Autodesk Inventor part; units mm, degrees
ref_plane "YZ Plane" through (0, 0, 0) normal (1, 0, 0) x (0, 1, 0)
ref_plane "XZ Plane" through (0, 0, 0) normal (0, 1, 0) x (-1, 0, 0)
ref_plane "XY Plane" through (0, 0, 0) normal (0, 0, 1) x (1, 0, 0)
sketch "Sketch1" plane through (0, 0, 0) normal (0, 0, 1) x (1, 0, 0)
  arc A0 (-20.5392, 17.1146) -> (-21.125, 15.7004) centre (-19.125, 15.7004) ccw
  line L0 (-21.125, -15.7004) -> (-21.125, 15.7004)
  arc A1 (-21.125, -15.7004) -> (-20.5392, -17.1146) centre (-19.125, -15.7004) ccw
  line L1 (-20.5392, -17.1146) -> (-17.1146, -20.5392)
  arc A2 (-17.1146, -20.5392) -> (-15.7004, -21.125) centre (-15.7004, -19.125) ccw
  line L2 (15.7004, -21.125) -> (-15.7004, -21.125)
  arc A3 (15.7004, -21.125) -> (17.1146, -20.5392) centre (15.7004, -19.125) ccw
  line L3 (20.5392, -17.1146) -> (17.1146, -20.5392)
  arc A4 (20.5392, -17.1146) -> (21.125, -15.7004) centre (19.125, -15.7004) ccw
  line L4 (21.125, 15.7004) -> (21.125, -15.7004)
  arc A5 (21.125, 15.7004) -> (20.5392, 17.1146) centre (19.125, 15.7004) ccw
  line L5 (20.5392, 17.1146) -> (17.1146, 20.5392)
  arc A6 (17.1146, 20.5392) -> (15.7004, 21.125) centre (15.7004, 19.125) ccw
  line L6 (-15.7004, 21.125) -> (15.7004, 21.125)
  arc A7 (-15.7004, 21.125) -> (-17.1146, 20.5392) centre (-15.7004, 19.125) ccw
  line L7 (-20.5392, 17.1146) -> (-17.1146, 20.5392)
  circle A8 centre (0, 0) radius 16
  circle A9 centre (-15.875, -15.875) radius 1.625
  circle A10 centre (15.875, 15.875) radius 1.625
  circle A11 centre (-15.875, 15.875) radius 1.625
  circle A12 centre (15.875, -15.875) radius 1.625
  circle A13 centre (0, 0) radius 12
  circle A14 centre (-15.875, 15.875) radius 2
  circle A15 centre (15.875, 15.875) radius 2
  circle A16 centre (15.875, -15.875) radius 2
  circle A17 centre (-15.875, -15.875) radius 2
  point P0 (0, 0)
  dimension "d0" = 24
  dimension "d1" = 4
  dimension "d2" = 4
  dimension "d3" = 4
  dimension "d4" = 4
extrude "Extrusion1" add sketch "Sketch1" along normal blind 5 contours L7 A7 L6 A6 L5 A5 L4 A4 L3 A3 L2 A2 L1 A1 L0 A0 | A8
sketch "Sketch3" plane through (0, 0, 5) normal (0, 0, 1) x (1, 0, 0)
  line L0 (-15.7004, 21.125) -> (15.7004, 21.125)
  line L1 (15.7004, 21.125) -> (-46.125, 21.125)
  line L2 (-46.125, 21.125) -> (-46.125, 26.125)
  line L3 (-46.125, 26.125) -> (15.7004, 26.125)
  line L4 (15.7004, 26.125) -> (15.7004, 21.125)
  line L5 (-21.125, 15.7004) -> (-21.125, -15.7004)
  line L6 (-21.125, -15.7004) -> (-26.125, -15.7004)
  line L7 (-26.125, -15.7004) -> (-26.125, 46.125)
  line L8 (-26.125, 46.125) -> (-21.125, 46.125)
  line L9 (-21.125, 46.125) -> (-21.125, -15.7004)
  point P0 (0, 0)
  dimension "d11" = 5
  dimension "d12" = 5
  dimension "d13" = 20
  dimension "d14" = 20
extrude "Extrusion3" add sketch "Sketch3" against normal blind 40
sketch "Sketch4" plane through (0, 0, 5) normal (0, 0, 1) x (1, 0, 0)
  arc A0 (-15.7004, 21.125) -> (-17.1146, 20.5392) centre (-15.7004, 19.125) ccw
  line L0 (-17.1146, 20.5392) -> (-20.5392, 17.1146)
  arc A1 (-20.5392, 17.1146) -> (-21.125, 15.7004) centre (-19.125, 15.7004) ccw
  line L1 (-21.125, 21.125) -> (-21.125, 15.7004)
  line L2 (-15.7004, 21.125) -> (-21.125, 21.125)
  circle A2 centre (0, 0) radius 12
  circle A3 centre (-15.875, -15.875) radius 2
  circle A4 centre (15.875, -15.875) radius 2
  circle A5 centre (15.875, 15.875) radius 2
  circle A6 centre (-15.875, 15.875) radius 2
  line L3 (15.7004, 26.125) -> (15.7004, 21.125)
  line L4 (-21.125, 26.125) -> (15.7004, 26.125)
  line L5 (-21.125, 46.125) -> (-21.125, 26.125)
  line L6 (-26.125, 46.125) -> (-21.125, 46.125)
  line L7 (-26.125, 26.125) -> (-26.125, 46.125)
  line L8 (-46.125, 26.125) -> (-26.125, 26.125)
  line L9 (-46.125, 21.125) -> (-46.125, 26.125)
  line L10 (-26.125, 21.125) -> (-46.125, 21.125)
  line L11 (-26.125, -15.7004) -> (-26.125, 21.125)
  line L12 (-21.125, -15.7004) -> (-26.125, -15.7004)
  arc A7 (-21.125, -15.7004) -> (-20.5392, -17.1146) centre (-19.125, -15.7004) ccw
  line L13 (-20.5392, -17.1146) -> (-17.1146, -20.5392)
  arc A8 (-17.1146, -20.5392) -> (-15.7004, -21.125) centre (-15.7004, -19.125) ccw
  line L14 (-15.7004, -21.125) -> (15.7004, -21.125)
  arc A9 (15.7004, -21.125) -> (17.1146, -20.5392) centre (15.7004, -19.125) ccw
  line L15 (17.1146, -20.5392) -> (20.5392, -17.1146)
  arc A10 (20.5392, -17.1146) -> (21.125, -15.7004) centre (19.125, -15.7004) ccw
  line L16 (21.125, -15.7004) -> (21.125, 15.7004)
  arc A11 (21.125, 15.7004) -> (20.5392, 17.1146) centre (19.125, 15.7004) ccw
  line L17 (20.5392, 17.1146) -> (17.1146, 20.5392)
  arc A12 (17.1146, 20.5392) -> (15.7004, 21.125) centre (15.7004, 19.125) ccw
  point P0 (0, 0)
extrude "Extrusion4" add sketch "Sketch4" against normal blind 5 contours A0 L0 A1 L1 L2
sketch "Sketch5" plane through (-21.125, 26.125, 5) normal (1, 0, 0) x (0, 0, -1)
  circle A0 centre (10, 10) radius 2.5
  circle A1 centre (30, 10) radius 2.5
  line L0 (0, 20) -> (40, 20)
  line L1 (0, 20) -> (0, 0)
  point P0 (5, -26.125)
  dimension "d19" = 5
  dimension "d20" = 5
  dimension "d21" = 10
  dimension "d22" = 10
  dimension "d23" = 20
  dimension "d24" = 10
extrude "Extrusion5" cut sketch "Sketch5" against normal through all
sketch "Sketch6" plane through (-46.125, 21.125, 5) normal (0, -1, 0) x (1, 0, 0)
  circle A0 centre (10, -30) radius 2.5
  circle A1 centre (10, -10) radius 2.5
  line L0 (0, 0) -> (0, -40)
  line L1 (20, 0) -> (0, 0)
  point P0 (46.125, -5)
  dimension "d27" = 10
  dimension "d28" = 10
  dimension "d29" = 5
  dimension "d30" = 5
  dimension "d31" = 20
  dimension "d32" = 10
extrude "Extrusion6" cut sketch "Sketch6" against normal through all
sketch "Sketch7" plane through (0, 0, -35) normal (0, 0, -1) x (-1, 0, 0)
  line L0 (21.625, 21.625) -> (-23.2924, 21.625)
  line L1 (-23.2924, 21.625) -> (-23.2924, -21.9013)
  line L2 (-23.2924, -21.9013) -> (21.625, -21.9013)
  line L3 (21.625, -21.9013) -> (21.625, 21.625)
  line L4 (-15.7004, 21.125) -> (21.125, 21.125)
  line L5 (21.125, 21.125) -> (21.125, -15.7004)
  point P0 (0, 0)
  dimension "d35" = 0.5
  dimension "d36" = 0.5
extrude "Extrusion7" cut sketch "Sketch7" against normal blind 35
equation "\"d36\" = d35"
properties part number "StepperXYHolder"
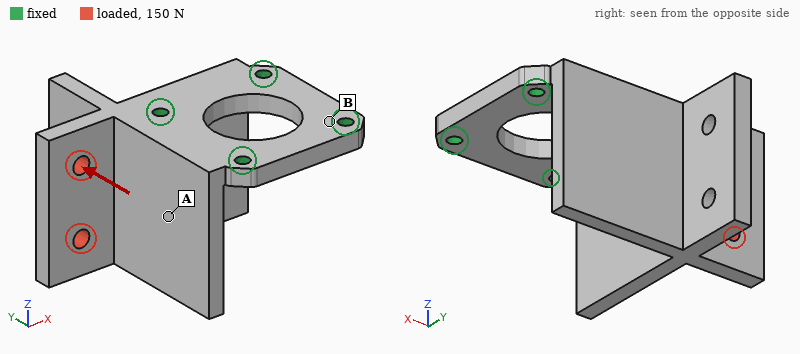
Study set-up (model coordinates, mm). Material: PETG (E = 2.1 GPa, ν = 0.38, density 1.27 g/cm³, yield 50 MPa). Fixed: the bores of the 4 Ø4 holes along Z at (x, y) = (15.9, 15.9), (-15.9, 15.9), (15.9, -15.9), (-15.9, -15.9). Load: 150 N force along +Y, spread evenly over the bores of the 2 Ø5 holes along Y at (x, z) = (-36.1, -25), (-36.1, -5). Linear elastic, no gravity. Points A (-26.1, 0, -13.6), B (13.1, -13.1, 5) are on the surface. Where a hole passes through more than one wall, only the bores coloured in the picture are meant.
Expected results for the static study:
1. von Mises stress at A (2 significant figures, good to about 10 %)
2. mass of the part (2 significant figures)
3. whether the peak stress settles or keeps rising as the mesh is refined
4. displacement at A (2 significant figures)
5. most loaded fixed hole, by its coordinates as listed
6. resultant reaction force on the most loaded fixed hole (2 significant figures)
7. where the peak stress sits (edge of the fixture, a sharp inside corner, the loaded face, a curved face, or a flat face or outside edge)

1.8 MPa
36 g
keeps rising
0.092 mm
(-15.9, -15.9)
140 N
a sharp inside corner
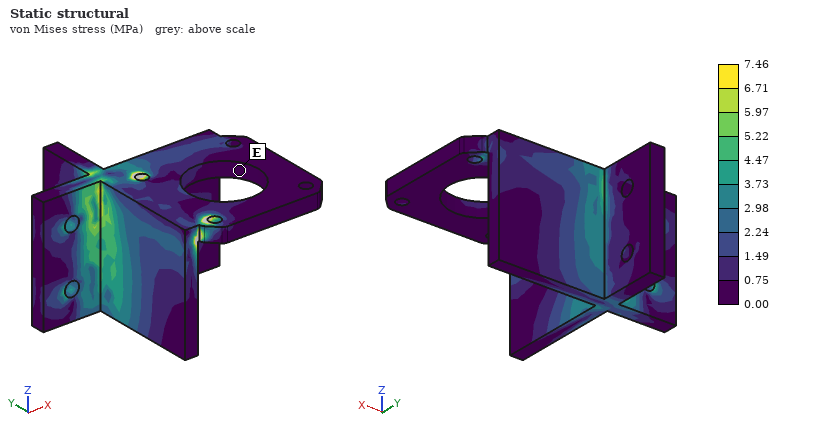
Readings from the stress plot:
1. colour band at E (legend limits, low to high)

0.00 to 0.75 MPa
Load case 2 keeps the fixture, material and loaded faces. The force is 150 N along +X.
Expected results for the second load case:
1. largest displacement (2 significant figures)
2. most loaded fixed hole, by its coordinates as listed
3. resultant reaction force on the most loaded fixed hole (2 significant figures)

0.18 mm
(-15.9, 15.9)
130 N
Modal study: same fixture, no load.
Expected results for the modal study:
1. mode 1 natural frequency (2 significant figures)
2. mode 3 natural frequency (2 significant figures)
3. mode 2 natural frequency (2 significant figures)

830 Hz
1300 Hz
940 Hz
